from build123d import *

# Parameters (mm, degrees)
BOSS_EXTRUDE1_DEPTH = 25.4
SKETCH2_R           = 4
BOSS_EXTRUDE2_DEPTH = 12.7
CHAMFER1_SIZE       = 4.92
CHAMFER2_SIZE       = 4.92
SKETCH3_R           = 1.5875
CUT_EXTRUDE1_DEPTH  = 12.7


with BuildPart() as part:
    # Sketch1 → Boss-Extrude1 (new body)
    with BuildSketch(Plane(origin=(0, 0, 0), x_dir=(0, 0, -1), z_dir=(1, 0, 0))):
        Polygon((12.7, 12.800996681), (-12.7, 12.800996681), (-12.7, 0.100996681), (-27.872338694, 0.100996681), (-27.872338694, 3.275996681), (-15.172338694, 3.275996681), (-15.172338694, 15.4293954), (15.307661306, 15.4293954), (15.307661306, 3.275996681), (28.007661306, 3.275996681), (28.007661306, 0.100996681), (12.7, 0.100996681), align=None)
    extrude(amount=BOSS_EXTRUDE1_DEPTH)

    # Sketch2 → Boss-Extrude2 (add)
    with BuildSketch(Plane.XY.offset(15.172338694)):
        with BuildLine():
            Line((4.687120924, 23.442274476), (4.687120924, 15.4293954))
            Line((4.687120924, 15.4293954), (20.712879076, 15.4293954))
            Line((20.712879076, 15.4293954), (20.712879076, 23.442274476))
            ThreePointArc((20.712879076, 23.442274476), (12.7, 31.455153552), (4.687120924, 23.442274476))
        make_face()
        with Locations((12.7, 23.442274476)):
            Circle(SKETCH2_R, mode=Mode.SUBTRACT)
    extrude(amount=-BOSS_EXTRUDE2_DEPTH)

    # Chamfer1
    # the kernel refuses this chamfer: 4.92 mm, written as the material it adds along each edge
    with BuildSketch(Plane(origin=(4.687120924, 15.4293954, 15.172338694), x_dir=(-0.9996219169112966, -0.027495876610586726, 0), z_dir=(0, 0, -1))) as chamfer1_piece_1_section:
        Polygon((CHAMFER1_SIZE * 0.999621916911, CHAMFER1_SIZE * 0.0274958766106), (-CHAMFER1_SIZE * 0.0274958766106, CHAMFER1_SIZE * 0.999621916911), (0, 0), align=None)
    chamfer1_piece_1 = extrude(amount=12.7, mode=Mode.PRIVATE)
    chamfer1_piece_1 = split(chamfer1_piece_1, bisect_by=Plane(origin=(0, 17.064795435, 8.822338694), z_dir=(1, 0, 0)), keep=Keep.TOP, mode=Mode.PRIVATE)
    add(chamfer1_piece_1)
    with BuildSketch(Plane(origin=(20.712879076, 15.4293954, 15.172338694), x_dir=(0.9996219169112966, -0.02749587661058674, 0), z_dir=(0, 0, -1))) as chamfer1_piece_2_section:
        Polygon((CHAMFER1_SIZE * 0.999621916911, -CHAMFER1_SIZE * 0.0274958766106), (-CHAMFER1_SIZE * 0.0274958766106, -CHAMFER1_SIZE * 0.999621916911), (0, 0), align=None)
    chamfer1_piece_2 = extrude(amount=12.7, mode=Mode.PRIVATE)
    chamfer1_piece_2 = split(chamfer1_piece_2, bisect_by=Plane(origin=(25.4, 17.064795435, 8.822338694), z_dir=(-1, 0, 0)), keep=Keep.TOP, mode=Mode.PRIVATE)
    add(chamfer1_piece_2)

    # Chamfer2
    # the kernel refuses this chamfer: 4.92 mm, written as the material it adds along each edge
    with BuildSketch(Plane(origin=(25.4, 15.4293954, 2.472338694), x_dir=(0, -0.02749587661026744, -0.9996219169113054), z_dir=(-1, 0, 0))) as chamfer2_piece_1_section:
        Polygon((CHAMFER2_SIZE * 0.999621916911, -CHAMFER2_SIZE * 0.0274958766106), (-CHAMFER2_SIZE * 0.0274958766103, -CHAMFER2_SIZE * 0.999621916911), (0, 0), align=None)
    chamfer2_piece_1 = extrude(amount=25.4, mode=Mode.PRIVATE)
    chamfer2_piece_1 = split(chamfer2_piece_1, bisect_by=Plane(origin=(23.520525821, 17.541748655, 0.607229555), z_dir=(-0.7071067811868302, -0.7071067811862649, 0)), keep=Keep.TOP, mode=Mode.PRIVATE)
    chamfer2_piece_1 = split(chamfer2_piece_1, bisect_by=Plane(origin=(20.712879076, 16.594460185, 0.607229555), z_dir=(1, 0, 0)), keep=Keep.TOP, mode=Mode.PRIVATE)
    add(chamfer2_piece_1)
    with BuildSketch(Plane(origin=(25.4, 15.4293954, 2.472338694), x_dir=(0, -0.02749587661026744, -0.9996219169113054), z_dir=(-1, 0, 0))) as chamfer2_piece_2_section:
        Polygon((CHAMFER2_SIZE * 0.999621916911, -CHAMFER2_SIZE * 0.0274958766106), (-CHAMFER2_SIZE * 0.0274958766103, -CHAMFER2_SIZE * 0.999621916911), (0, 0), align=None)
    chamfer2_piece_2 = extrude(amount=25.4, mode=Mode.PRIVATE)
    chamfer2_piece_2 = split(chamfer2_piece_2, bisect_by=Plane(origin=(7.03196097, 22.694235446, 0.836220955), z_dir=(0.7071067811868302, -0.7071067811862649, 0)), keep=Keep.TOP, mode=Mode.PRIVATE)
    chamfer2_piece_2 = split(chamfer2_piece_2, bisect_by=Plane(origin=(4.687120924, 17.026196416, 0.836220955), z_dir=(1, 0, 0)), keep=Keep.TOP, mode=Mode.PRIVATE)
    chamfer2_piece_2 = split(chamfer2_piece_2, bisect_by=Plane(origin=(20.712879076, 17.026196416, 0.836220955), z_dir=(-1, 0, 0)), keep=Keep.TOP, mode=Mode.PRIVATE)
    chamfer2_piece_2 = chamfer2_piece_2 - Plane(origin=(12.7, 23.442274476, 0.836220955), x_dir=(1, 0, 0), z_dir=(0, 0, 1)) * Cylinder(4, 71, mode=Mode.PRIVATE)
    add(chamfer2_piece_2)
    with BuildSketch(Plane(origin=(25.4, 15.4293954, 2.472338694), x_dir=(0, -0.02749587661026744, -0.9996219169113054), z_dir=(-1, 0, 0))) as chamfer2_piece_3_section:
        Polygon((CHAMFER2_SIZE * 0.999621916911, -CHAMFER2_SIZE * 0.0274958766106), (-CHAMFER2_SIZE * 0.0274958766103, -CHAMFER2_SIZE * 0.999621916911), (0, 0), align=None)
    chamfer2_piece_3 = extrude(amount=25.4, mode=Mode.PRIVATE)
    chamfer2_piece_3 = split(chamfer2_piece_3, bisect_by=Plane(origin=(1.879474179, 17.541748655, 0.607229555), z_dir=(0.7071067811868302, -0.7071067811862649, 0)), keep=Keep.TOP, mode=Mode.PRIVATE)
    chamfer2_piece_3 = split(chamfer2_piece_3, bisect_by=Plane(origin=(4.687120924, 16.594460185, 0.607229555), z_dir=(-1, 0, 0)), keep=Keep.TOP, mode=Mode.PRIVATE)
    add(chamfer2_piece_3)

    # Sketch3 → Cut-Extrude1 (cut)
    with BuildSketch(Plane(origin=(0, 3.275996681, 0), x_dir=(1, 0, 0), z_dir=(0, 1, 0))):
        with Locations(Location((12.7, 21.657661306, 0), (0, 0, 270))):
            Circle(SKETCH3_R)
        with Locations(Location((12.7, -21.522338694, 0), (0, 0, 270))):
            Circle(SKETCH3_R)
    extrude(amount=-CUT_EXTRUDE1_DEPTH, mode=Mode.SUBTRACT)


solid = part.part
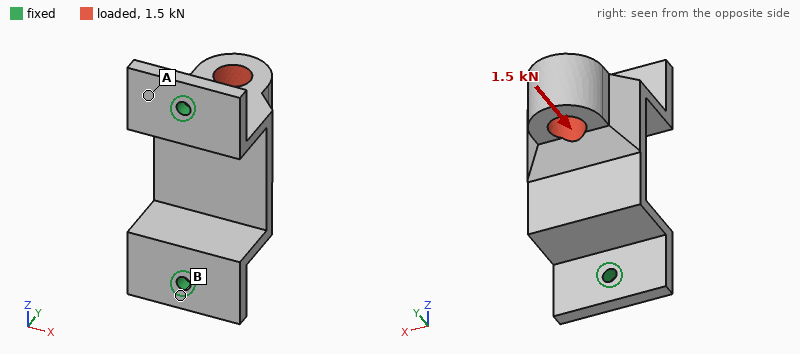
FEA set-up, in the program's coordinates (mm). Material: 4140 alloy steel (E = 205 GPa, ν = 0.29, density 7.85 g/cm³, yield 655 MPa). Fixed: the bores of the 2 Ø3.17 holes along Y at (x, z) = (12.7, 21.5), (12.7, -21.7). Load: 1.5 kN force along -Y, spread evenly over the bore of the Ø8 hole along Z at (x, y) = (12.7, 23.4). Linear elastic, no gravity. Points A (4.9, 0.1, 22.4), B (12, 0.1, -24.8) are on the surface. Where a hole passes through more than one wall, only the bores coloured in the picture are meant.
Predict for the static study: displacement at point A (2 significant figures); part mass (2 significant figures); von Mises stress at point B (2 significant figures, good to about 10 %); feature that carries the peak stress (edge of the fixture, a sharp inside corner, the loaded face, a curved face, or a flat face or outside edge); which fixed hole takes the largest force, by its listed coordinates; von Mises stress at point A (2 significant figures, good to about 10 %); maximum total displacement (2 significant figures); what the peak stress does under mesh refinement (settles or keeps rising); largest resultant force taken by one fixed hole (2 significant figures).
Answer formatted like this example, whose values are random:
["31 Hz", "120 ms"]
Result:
["2.9 µm", "67 g", "16 MPa", "edge of the fixture", "(12.7, 21.5)", "31 MPa", "16 µm", "keeps rising", "1.2 kN"]
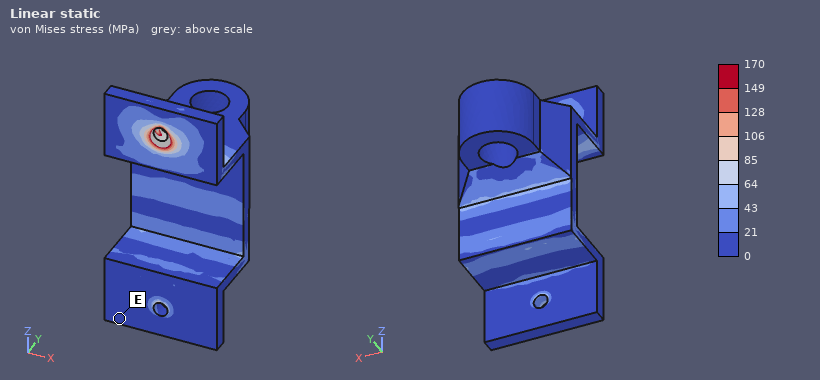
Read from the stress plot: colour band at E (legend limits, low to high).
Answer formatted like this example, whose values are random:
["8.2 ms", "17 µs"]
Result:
["0 to 21 MPa"]
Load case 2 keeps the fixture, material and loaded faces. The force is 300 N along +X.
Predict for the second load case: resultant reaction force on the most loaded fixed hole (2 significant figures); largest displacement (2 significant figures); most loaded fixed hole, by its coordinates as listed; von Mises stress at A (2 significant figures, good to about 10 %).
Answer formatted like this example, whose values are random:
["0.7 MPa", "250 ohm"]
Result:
["200 N", "51 µm", "(12.7, 21.5)", "37 MPa"]
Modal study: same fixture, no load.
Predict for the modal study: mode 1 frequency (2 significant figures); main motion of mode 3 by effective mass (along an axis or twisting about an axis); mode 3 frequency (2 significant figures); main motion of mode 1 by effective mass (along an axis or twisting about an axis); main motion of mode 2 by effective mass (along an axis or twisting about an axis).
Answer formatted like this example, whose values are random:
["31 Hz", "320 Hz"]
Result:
["2700 Hz", "along Y", "8200 Hz", "along X", "along Z"]
